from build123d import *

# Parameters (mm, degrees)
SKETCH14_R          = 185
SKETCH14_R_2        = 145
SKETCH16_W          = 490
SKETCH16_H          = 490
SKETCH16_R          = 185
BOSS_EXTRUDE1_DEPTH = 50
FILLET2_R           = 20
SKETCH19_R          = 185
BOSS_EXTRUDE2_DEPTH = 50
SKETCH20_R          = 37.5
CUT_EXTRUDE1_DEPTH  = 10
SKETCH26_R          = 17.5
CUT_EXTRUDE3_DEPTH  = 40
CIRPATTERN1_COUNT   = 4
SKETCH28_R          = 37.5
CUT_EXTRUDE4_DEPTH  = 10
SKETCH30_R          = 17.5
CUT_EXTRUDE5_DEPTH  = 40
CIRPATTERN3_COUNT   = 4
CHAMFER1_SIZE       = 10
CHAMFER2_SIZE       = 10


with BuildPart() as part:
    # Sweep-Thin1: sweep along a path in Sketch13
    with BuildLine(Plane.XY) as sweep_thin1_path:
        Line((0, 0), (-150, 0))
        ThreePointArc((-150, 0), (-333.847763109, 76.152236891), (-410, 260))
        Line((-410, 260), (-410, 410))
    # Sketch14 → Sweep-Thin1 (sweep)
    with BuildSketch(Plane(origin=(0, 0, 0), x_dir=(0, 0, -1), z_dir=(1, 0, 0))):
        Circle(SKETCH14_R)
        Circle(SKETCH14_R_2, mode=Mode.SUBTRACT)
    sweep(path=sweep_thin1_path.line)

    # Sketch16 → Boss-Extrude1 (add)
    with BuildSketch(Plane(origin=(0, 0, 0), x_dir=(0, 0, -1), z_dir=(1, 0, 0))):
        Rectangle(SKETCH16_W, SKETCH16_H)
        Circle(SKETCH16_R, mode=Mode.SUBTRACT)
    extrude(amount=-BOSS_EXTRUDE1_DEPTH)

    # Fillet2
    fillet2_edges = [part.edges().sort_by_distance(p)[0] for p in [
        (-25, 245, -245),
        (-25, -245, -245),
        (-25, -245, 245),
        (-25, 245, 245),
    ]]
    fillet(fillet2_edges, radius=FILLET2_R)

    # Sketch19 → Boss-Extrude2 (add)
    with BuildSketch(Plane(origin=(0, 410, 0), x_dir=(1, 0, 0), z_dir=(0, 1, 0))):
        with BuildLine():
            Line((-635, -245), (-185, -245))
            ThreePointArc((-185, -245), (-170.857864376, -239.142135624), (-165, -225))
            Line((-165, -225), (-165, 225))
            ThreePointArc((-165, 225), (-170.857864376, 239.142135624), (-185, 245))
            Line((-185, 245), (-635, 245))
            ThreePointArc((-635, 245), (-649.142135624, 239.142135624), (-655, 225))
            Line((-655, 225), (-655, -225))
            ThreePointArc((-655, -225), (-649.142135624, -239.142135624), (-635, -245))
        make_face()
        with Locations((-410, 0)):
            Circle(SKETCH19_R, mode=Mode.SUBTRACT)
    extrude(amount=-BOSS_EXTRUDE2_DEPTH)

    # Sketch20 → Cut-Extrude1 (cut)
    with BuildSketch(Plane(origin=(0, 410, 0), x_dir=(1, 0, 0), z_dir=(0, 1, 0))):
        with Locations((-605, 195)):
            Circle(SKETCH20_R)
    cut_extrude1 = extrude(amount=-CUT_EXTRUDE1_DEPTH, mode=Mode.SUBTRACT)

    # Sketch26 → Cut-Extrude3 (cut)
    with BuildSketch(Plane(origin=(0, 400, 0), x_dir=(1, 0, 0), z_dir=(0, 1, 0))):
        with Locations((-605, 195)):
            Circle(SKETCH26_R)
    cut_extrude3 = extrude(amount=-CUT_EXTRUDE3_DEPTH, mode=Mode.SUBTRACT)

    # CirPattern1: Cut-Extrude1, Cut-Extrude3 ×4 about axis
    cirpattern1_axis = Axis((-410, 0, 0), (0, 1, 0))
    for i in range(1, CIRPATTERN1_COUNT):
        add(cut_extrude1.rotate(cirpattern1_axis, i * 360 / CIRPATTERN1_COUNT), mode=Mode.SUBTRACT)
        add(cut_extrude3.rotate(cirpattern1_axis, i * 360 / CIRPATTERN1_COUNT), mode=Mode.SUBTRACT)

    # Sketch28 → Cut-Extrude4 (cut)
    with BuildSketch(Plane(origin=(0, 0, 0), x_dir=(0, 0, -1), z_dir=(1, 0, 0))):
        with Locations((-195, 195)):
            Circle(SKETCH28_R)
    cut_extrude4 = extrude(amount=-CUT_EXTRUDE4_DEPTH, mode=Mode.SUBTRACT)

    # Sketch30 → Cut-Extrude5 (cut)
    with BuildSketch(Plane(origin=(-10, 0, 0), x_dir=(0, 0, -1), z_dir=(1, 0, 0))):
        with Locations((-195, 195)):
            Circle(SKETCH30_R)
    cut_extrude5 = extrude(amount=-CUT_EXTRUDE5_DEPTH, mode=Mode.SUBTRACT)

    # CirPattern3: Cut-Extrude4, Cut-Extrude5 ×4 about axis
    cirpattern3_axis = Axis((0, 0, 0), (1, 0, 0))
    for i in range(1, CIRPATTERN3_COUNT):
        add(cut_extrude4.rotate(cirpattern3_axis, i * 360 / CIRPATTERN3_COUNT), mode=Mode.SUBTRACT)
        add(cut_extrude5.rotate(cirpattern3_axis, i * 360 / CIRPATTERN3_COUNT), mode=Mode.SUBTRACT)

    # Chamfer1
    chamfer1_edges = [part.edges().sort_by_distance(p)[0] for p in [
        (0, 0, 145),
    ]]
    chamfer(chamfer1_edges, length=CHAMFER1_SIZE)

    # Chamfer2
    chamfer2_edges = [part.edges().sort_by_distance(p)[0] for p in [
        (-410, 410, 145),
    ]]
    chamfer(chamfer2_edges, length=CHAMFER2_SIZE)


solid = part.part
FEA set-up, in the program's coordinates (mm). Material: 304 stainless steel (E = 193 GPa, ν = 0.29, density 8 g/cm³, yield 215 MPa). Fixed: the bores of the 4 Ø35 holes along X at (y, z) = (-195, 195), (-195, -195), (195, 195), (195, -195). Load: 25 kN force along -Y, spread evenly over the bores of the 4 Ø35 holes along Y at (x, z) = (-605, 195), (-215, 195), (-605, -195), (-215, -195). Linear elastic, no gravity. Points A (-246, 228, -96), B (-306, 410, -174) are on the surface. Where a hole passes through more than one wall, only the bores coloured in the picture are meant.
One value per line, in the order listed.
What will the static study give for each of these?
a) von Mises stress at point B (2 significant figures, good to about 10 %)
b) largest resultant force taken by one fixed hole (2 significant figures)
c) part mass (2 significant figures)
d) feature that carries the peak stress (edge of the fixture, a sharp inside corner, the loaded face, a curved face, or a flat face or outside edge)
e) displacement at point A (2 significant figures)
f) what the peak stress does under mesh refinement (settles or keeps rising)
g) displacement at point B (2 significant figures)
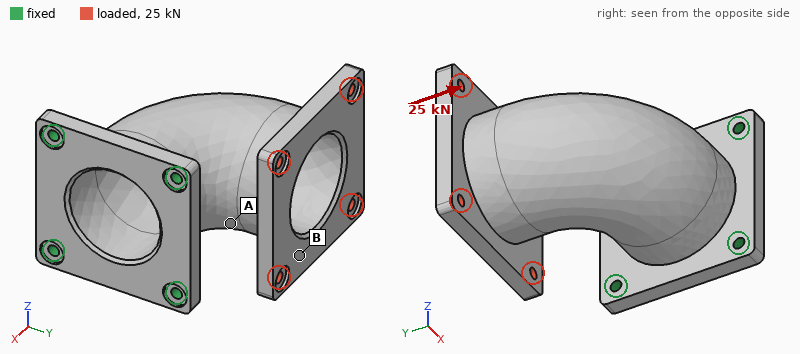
4.2 MPa
15 kN
330 kg
edge of the fixture
0.032 mm
keeps rising
0.055 mm
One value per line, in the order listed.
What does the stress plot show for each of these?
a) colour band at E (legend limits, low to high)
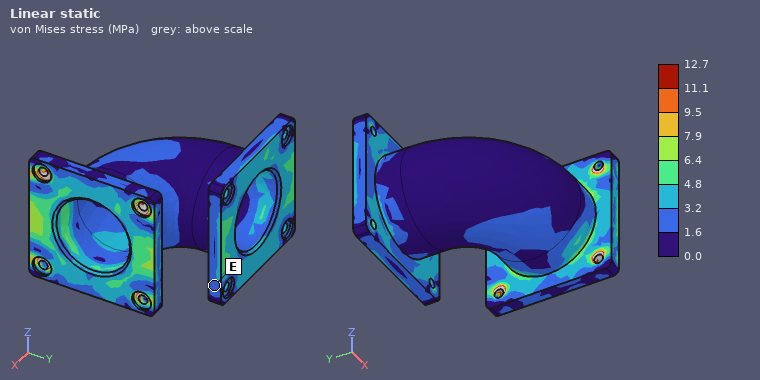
1.6 to 3.2 MPa
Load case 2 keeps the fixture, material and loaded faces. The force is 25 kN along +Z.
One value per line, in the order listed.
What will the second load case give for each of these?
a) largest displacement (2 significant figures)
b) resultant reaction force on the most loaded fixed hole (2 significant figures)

0.11 mm
18 kN
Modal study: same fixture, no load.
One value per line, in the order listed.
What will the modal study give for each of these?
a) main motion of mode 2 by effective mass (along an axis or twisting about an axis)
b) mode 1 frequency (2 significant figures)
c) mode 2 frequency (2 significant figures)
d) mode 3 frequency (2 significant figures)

along Z
200 Hz
230 Hz
560 Hz
